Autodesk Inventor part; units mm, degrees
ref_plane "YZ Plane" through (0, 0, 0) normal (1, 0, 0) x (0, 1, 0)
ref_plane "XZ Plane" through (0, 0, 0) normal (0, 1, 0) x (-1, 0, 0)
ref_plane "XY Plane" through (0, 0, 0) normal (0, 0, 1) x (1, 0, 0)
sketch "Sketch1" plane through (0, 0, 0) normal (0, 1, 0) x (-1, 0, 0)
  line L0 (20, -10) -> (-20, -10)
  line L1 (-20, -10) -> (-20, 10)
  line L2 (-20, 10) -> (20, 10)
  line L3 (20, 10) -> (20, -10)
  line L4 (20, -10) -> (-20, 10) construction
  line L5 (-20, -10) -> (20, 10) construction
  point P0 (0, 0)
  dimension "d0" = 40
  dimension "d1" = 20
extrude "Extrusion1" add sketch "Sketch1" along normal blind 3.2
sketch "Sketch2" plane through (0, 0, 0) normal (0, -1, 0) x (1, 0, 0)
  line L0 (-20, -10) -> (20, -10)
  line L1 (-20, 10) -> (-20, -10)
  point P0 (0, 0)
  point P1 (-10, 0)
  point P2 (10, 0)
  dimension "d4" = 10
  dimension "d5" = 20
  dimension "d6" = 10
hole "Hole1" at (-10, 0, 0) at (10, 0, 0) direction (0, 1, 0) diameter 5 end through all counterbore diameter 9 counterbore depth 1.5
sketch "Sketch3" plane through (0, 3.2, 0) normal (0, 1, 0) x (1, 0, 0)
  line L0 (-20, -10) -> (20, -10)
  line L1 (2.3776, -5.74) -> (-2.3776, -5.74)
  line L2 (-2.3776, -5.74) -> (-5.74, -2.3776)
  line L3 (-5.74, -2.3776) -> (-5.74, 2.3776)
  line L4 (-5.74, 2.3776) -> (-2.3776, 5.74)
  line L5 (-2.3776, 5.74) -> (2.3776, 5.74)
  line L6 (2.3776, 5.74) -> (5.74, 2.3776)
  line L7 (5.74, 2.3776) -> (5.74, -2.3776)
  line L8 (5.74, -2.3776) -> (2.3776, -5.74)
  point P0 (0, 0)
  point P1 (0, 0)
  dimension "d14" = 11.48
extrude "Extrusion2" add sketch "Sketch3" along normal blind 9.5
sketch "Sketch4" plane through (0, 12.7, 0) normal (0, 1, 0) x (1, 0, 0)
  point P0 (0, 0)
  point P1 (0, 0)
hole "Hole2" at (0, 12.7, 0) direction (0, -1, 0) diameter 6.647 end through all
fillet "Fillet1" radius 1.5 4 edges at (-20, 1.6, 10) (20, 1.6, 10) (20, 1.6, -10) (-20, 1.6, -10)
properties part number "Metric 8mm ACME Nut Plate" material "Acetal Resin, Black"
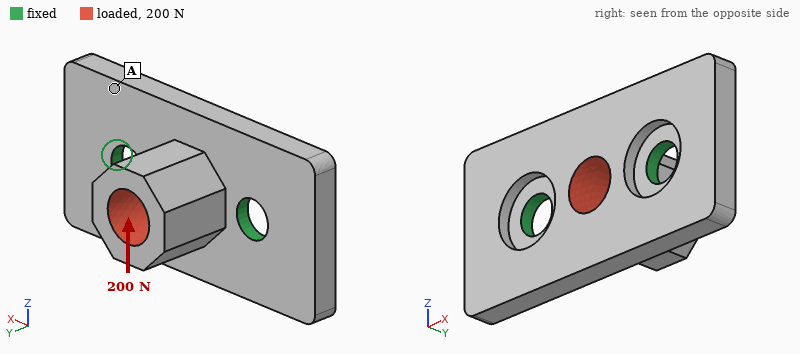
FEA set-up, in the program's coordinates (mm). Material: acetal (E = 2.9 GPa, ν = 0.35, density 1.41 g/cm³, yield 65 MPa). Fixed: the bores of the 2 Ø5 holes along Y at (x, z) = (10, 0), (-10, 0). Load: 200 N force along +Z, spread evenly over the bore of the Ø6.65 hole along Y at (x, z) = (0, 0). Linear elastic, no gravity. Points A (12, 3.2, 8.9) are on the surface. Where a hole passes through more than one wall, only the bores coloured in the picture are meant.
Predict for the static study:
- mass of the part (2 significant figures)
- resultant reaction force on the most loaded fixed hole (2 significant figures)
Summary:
4.1 g
100 N
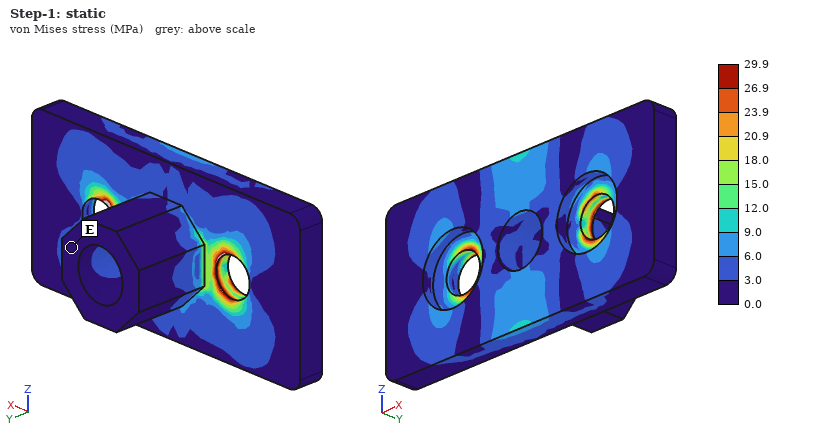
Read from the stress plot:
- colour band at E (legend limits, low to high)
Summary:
0.0 to 3.0 MPa
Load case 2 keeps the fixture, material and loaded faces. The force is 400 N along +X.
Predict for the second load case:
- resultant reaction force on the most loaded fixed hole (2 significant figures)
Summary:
230 N
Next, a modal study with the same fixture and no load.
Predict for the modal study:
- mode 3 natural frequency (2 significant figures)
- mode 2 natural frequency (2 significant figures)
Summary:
5100 Hz
5000 Hz
